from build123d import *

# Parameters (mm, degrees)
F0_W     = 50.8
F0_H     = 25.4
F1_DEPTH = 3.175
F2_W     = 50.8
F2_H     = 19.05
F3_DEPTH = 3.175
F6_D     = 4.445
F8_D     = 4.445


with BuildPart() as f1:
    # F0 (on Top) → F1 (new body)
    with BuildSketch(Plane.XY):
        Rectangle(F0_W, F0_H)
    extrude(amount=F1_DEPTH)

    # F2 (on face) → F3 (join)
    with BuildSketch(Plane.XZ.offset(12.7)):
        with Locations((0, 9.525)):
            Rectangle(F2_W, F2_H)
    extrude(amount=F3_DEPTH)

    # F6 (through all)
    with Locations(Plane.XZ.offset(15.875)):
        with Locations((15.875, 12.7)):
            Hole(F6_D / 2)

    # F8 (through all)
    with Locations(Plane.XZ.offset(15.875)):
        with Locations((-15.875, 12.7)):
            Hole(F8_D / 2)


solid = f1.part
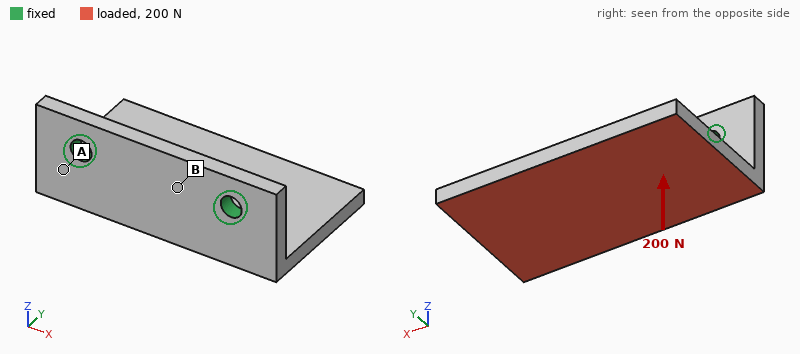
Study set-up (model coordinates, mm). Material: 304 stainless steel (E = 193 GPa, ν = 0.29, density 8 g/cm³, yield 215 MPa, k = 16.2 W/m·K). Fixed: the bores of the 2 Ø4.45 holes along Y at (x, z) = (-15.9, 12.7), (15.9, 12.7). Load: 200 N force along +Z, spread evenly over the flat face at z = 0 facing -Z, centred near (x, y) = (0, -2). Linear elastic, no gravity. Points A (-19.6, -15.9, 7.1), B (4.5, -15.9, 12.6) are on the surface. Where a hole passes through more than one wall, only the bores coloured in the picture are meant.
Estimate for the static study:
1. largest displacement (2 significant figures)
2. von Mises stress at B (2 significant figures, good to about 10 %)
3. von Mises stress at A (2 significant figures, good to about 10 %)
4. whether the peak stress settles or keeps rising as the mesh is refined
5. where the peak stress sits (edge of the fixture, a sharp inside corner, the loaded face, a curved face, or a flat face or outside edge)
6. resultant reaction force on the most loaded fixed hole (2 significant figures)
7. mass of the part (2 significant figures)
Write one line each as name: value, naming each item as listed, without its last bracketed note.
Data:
largest displacement: 44 µm
von Mises stress at B: 11 MPa
von Mises stress at A: 29 MPa
whether the peak stress settles or keeps rising as the mesh is refined: keeps rising
where the peak stress sits: edge of the fixture
resultant reaction force on the most loaded fixed hole: 100 N
mass of the part: 57 g
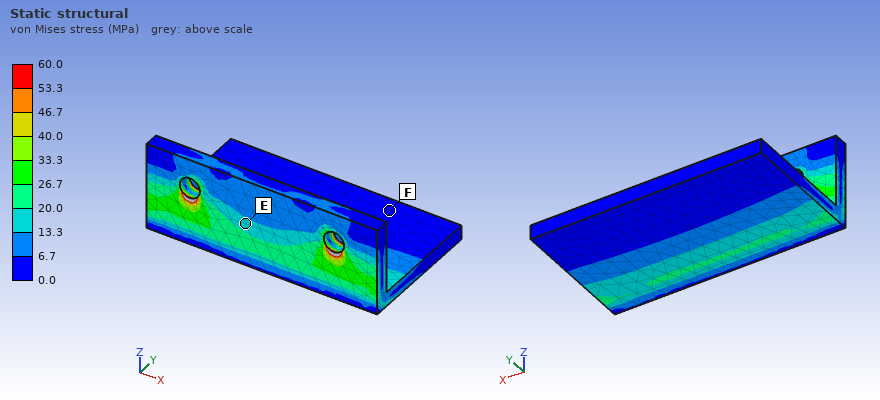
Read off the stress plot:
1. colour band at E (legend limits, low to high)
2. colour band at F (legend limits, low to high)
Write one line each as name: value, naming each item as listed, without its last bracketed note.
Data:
colour band at E: 13.3 to 20.0 MPa
colour band at F: 0.0 to 6.7 MPa
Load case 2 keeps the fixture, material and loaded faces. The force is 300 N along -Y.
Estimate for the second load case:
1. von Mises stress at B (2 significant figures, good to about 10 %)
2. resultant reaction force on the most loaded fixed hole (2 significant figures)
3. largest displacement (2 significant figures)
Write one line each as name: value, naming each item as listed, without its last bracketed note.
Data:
von Mises stress at B: 11 MPa
resultant reaction force on the most loaded fixed hole: 150 N
largest displacement: 30 µm
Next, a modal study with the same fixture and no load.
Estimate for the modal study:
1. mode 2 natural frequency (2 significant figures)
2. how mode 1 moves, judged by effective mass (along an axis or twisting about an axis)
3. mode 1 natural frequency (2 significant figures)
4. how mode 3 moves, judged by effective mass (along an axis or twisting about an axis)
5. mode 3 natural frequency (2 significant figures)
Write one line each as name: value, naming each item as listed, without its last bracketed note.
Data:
mode 2 natural frequency: 4100 Hz
how mode 1 moves, judged by effective mass: along Z
mode 1 natural frequency: 2100 Hz
how mode 3 moves, judged by effective mass: along X
mode 3 natural frequency: 6900 Hz
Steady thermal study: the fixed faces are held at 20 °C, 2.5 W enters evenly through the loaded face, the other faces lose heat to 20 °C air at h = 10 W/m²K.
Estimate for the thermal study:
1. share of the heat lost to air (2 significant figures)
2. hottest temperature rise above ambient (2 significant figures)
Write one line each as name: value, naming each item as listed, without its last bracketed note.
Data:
share of the heat lost to air: 16 %
hottest temperature rise above ambient: 21 K
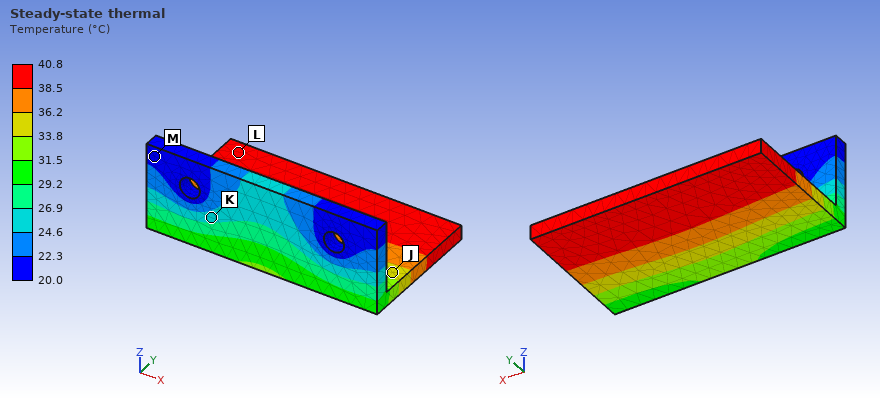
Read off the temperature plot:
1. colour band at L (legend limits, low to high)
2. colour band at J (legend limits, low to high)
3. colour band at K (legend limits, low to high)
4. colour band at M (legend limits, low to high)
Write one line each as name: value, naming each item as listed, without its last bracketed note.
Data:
colour band at L: 38.5 to 40.8 °C
colour band at J: 33.8 to 36.2 °C
colour band at K: 24.6 to 26.9 °C
colour band at M: 20.0 to 22.3 °C
